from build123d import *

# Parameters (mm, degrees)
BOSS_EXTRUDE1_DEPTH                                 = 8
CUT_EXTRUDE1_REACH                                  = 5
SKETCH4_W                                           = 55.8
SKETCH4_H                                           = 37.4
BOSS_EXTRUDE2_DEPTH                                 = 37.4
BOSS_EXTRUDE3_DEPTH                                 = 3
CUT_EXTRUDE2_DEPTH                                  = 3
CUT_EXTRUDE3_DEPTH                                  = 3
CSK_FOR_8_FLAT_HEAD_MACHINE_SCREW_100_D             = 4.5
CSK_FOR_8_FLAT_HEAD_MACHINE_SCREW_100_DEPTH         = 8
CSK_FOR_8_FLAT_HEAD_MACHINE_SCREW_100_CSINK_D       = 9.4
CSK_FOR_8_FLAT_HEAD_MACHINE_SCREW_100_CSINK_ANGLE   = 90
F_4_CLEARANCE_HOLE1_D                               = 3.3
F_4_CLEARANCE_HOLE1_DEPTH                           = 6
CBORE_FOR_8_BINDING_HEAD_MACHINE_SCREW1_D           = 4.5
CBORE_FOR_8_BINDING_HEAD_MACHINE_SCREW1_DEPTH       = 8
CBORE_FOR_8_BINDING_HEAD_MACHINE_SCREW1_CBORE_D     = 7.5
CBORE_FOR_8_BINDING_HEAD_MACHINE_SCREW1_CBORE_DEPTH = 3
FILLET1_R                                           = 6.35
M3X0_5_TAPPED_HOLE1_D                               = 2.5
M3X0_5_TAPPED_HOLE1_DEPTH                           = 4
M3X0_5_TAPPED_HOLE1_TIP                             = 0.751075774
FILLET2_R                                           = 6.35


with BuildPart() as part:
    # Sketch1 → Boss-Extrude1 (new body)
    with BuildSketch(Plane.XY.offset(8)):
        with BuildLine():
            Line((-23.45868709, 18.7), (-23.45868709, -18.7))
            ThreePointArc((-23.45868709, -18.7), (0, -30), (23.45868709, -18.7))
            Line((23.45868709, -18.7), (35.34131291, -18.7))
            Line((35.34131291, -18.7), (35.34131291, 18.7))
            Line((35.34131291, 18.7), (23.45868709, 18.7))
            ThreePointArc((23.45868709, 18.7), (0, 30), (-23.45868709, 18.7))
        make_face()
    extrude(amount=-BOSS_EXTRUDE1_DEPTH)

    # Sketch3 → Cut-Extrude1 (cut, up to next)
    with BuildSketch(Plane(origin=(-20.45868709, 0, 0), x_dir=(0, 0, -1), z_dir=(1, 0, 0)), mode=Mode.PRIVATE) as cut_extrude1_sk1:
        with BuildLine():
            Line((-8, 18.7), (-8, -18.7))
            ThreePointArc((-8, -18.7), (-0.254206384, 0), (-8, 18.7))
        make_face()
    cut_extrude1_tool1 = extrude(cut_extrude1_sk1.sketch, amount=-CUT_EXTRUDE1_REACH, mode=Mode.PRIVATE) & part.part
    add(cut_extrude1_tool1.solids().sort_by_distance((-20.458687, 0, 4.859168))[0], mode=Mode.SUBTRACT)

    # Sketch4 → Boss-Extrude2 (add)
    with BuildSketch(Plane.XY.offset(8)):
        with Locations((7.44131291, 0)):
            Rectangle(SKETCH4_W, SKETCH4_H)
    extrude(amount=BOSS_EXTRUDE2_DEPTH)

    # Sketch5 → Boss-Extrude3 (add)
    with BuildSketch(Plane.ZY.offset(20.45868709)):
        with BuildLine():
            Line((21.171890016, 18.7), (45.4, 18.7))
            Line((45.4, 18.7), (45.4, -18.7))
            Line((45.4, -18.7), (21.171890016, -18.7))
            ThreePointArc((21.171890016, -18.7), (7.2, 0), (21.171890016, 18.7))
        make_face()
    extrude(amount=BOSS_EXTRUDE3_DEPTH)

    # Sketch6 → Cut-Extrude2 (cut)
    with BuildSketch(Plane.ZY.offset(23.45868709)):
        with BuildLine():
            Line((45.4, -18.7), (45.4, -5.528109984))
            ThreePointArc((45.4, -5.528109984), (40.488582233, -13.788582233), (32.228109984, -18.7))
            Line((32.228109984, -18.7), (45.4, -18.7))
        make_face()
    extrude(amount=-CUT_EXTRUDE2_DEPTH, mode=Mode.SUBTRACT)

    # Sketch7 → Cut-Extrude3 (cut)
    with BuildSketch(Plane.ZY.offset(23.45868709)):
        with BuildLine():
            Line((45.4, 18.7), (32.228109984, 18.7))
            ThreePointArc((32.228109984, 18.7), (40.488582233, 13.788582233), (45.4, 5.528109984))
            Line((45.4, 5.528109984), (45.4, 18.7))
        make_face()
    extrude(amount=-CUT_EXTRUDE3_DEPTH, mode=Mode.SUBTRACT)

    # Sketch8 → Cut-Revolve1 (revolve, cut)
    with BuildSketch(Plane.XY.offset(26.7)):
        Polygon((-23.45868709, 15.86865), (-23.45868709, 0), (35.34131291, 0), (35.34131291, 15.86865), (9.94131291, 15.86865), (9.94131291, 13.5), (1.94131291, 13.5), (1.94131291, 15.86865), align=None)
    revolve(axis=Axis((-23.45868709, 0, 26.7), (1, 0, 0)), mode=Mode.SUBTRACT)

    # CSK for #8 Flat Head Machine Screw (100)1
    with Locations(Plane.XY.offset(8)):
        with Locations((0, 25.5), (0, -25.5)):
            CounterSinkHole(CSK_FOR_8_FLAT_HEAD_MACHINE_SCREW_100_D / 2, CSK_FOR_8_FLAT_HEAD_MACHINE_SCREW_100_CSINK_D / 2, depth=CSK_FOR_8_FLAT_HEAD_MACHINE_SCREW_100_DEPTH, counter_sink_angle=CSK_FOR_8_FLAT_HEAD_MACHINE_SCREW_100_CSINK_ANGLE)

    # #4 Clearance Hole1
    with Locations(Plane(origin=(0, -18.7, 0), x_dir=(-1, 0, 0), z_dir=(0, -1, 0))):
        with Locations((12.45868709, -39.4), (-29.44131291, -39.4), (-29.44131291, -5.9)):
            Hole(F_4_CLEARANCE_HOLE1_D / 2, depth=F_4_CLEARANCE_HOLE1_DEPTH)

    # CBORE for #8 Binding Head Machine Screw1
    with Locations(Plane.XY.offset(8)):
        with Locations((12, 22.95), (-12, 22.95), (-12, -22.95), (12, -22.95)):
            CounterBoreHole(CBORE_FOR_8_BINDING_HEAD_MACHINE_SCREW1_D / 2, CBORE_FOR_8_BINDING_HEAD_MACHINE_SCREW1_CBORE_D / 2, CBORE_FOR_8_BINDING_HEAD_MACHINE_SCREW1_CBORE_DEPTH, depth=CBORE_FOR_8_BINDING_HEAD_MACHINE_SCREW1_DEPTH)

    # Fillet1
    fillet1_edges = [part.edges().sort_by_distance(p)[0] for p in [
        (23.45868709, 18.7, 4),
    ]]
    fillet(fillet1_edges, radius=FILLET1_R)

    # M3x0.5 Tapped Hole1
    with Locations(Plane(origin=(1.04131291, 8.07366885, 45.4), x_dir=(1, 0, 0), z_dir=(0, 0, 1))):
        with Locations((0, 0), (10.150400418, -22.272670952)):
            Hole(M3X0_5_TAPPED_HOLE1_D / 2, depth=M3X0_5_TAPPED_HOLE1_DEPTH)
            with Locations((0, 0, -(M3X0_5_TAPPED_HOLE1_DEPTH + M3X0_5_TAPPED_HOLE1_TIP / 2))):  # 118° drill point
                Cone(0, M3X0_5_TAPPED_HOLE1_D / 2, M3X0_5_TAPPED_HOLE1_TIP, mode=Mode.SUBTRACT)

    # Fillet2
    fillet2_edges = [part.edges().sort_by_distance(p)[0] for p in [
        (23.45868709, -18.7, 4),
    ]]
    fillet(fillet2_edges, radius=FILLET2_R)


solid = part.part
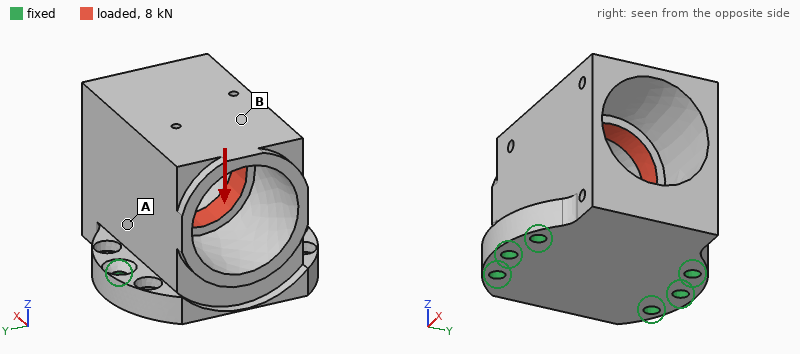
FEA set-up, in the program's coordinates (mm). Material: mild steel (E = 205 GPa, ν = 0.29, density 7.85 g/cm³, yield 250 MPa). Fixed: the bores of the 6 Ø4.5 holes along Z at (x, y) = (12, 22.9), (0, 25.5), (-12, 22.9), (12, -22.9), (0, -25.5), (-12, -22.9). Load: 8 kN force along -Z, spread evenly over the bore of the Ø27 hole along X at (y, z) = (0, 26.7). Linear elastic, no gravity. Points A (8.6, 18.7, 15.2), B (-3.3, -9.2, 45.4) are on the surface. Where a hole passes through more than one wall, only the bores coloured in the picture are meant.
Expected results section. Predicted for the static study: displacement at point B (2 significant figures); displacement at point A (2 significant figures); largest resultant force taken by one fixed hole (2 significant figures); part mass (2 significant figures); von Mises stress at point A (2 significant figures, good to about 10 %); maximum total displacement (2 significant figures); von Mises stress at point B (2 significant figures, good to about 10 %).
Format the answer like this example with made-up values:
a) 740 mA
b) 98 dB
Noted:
a) 7.7 µm
b) 4.2 µm
c) 2.6 kN
d) 460 g
e) 35 MPa
f) 11 µm
g) 10 MPa
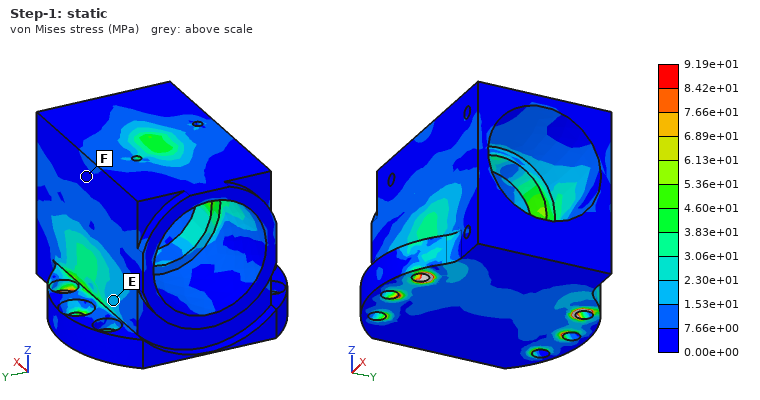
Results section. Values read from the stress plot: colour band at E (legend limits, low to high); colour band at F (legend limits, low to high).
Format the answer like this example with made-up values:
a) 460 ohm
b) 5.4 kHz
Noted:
a) 1.53e+01 to 2.30e+01 MPa
b) 0.00e+00 to 7.66e+00 MPa
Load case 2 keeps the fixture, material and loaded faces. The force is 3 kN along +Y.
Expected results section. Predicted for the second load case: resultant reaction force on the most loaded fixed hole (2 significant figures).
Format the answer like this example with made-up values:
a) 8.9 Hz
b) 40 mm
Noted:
a) 990 N
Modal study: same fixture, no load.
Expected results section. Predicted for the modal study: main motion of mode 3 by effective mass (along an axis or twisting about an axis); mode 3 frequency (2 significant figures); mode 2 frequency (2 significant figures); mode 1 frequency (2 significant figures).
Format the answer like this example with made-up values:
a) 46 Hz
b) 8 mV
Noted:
a) twisting about Z
b) 8400 Hz
c) 4900 Hz
d) 4800 Hz
